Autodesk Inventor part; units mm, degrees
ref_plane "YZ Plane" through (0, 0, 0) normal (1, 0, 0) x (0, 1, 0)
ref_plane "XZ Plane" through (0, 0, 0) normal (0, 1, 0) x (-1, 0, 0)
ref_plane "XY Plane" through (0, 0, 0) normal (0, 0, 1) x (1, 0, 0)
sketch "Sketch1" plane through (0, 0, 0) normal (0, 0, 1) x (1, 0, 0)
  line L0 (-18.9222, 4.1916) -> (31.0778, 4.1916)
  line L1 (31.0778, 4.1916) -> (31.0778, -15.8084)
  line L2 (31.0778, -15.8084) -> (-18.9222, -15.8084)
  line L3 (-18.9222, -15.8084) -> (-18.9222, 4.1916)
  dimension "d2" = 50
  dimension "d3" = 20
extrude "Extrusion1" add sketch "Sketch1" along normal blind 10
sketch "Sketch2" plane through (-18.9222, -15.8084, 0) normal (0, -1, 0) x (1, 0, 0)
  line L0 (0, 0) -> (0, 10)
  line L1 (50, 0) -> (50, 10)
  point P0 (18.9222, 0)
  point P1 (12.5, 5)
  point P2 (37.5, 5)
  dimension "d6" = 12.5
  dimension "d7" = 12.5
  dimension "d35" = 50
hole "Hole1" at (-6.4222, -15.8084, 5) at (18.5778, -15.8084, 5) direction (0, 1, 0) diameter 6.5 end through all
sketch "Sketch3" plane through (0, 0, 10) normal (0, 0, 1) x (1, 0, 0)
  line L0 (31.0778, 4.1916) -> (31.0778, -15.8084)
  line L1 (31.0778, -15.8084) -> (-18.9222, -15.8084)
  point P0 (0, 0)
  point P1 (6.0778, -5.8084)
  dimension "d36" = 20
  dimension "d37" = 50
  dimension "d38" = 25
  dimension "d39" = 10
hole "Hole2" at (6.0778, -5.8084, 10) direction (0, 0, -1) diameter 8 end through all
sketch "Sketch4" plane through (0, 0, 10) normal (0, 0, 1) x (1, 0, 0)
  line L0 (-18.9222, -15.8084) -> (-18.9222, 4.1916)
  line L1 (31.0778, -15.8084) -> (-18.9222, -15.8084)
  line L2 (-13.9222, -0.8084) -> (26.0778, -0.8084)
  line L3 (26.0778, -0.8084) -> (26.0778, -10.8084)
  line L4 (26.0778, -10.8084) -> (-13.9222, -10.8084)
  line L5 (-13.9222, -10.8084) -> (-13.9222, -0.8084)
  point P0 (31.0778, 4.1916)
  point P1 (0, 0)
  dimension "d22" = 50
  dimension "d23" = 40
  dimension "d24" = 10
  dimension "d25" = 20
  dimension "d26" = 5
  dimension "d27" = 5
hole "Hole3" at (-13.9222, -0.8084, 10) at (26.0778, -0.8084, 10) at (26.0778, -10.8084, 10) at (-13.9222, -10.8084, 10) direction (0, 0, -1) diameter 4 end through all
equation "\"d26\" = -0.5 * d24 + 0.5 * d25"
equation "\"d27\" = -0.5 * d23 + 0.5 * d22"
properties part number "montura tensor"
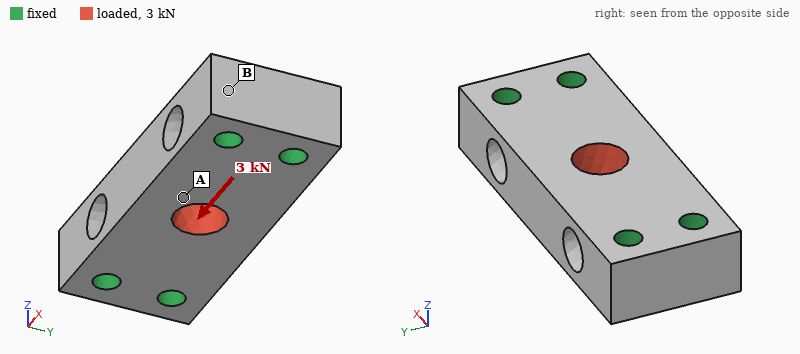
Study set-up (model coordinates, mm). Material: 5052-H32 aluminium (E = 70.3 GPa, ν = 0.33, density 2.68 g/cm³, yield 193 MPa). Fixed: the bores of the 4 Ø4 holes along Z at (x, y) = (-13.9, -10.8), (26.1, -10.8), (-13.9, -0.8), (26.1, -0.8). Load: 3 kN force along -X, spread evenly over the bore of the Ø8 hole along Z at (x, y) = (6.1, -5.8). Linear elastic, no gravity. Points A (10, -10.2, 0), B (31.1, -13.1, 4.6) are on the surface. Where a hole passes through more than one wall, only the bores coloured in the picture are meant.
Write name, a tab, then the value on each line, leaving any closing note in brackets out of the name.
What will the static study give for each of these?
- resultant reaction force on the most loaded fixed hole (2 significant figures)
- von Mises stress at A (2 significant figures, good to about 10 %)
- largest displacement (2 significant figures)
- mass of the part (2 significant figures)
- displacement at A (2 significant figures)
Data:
resultant reaction force on the most loaded fixed hole	760 N
von Mises stress at A	12 MPa
largest displacement	4.1 µm
mass of the part	21 g
displacement at A	3.5 µm
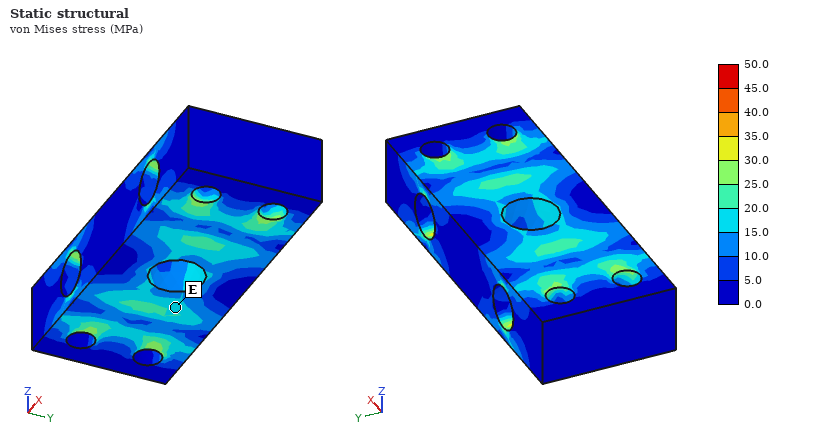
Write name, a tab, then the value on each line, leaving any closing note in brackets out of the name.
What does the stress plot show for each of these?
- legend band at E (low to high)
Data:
legend band at E	15.0 to 20.0 MPa
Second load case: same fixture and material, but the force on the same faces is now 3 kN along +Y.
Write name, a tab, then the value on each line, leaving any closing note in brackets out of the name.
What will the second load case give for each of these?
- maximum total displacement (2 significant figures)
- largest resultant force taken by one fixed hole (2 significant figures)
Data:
maximum total displacement	12 µm
largest resultant force taken by one fixed hole	1.1 kN
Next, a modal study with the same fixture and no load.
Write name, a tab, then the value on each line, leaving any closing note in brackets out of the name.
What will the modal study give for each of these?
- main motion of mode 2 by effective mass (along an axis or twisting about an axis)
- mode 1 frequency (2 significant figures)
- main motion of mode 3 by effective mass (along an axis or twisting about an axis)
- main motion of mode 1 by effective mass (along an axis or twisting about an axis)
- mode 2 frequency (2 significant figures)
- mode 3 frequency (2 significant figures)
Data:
main motion of mode 2 by effective mass	twisting about X
mode 1 frequency	17 kHz
main motion of mode 3 by effective mass	along Y
main motion of mode 1 by effective mass	along Z
mode 2 frequency	25 kHz
mode 3 frequency	29 kHz
